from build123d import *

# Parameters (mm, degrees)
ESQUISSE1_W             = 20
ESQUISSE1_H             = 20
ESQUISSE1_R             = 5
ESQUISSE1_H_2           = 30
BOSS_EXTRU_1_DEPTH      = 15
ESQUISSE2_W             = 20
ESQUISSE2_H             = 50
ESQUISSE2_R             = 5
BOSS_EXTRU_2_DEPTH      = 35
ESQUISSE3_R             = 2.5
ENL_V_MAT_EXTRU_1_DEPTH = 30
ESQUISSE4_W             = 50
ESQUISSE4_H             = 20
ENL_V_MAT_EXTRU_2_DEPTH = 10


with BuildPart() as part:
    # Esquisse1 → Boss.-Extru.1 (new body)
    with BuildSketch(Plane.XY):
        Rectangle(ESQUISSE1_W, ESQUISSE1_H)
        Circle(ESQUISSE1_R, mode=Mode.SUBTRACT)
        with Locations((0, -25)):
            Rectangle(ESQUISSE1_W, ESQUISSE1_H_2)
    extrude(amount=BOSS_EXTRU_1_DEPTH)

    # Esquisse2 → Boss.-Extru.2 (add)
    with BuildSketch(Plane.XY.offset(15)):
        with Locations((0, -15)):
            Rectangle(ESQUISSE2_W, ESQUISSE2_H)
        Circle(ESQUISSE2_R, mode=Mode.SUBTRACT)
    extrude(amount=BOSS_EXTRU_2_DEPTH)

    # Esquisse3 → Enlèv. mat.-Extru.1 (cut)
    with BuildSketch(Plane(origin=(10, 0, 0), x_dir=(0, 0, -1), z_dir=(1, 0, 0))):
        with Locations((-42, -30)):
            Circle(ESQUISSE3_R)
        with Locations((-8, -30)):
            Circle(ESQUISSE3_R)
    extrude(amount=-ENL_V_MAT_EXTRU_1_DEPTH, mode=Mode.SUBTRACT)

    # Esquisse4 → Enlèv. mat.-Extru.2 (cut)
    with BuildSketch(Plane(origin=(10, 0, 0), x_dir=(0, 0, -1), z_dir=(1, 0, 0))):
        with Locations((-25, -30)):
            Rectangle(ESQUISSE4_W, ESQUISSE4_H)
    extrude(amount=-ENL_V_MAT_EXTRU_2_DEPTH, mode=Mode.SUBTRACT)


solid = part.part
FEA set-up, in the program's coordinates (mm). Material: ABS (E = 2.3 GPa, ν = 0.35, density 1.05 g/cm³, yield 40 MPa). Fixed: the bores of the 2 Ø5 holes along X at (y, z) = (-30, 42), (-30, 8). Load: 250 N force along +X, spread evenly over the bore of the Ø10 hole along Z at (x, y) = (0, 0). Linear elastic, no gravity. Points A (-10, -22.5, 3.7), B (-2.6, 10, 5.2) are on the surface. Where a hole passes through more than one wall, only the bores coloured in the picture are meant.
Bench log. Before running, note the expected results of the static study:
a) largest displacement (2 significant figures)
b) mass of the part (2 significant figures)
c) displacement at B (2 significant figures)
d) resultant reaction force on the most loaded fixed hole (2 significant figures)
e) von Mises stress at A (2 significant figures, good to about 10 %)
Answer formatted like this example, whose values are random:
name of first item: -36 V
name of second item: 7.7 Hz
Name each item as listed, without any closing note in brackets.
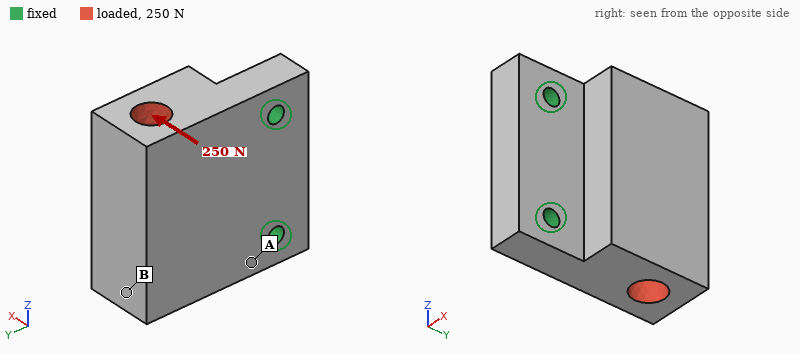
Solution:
largest displacement: 0.40 mm
mass of the part: 37 g
displacement at B: 0.37 mm
resultant reaction force on the most loaded fixed hole: 130 N
von Mises stress at A: 7.0 MPa
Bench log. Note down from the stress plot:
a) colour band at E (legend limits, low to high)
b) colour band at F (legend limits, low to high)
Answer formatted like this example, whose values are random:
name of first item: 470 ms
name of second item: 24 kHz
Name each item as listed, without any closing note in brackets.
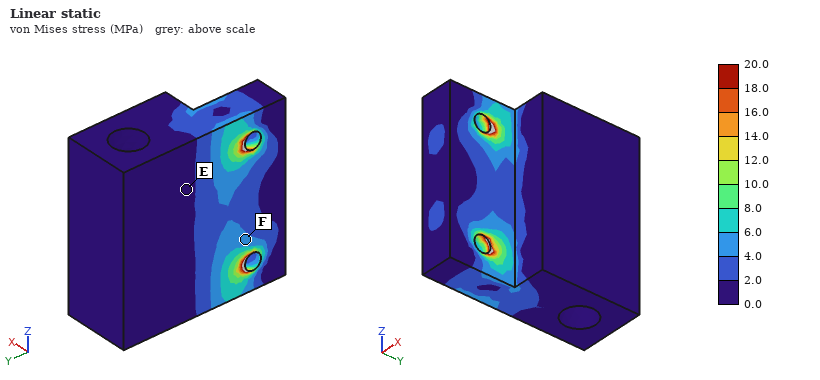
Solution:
colour band at E: 0.0 to 2.0 MPa
colour band at F: 4.0 to 6.0 MPa
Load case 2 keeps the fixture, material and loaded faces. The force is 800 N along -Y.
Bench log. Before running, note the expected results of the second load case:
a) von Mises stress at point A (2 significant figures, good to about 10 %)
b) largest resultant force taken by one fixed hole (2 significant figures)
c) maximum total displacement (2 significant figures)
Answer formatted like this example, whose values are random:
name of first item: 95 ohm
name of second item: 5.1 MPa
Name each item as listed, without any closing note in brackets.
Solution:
von Mises stress at point A: 3.0 MPa
largest resultant force taken by one fixed hole: 400 N
maximum total displacement: 0.25 mm
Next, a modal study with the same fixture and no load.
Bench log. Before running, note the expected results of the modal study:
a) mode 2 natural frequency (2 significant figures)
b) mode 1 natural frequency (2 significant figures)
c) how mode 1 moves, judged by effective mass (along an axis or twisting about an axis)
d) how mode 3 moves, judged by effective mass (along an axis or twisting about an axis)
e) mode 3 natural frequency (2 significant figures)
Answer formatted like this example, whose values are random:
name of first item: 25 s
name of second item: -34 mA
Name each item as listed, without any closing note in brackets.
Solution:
mode 2 natural frequency: 2900 Hz
mode 1 natural frequency: 1000 Hz
how mode 1 moves, judged by effective mass: along X
how mode 3 moves, judged by effective mass: along Z
mode 3 natural frequency: 3200 Hz
